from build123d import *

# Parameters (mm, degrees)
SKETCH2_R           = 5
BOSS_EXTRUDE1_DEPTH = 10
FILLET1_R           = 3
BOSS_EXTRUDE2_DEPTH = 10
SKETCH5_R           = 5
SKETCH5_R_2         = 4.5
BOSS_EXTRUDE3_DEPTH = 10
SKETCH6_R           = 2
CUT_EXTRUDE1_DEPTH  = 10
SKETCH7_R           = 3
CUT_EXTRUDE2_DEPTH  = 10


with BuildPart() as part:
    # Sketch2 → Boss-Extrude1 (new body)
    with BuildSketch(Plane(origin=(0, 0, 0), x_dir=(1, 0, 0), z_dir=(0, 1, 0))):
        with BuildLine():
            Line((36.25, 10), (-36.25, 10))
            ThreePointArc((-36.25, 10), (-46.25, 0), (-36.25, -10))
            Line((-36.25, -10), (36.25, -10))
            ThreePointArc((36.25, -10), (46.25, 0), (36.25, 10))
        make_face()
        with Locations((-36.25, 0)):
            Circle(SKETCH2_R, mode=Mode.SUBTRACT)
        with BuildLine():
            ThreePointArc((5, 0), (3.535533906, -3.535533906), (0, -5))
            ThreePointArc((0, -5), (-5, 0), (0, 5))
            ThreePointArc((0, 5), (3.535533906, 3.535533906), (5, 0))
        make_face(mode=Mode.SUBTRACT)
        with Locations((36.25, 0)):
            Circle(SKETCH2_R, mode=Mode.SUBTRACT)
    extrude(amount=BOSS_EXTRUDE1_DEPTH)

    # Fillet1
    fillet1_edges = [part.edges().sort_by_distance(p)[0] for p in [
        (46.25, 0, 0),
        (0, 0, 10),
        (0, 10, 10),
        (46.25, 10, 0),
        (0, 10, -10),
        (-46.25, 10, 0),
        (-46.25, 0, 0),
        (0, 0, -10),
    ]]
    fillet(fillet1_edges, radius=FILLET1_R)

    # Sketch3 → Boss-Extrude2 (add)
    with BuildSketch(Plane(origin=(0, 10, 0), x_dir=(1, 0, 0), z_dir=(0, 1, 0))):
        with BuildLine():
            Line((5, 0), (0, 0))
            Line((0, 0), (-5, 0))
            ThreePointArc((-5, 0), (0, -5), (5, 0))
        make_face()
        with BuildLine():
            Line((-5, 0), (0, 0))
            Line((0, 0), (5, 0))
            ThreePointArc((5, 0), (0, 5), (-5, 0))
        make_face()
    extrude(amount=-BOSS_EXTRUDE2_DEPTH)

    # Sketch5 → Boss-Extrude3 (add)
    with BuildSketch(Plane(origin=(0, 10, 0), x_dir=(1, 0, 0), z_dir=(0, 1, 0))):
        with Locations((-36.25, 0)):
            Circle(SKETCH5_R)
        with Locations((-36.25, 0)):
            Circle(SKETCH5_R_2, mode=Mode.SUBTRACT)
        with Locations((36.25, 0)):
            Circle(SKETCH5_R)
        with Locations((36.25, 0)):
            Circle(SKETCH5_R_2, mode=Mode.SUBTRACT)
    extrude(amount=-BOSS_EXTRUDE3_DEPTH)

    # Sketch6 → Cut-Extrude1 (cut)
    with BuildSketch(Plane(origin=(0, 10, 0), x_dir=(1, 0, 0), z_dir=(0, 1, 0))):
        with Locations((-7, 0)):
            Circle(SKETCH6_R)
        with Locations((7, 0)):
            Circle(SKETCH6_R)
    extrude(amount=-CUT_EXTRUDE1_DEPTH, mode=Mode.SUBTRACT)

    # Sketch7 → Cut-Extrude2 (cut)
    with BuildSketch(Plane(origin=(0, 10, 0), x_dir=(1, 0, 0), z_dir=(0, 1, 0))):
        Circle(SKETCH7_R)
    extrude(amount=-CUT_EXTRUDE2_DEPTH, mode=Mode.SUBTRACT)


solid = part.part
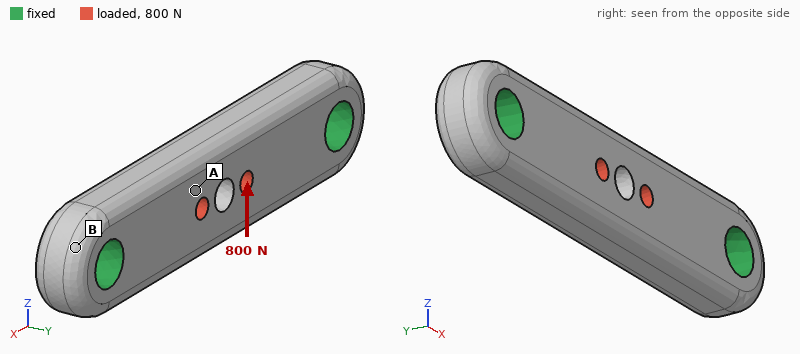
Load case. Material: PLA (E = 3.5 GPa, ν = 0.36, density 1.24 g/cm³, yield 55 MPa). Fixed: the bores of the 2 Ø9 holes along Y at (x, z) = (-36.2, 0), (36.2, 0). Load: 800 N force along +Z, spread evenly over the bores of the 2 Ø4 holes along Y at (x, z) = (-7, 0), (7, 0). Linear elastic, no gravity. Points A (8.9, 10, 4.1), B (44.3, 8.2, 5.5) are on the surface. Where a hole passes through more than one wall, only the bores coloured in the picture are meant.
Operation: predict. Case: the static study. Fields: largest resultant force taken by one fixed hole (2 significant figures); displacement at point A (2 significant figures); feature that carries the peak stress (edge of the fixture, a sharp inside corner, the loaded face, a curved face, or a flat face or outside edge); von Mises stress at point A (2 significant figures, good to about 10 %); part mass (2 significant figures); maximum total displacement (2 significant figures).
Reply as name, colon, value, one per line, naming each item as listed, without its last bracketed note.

largest resultant force taken by one fixed hole: 400 N
displacement at point A: 0.12 mm
feature that carries the peak stress: edge of the fixture
von Mises stress at point A: 5.1 MPa
part mass: 19 g
maximum total displacement: 0.13 mm
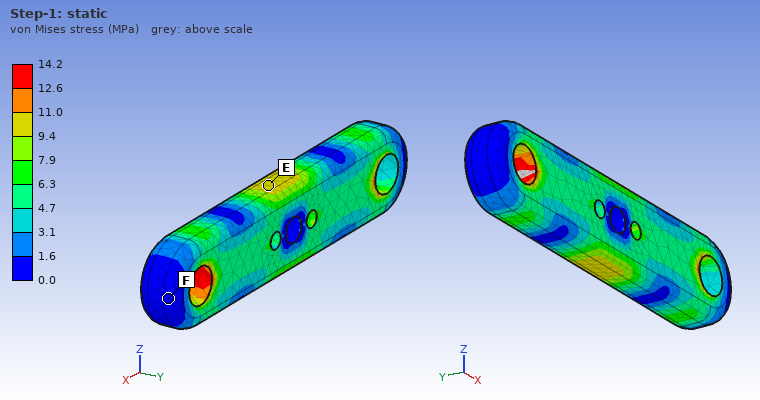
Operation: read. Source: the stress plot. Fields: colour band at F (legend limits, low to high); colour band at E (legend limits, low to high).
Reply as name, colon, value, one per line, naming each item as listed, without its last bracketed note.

colour band at F: 0.0 to 1.6 MPa
colour band at E: 9.4 to 11.0 MPa
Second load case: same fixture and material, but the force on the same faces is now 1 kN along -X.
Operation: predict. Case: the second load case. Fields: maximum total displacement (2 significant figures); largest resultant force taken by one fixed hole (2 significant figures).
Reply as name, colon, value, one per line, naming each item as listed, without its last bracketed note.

maximum total displacement: 30 µm
largest resultant force taken by one fixed hole: 500 N
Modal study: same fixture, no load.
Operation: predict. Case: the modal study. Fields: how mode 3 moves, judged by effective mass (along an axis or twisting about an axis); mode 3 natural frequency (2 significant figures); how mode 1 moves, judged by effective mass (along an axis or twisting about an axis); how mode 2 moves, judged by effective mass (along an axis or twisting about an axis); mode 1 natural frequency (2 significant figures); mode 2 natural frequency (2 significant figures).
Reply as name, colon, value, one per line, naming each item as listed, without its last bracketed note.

how mode 3 moves, judged by effective mass: twisting about X
mode 3 natural frequency: 6000 Hz
how mode 1 moves, judged by effective mass: along Y
how mode 2 moves, judged by effective mass: along Z
mode 1 natural frequency: 3400 Hz
mode 2 natural frequency: 4700 Hz
